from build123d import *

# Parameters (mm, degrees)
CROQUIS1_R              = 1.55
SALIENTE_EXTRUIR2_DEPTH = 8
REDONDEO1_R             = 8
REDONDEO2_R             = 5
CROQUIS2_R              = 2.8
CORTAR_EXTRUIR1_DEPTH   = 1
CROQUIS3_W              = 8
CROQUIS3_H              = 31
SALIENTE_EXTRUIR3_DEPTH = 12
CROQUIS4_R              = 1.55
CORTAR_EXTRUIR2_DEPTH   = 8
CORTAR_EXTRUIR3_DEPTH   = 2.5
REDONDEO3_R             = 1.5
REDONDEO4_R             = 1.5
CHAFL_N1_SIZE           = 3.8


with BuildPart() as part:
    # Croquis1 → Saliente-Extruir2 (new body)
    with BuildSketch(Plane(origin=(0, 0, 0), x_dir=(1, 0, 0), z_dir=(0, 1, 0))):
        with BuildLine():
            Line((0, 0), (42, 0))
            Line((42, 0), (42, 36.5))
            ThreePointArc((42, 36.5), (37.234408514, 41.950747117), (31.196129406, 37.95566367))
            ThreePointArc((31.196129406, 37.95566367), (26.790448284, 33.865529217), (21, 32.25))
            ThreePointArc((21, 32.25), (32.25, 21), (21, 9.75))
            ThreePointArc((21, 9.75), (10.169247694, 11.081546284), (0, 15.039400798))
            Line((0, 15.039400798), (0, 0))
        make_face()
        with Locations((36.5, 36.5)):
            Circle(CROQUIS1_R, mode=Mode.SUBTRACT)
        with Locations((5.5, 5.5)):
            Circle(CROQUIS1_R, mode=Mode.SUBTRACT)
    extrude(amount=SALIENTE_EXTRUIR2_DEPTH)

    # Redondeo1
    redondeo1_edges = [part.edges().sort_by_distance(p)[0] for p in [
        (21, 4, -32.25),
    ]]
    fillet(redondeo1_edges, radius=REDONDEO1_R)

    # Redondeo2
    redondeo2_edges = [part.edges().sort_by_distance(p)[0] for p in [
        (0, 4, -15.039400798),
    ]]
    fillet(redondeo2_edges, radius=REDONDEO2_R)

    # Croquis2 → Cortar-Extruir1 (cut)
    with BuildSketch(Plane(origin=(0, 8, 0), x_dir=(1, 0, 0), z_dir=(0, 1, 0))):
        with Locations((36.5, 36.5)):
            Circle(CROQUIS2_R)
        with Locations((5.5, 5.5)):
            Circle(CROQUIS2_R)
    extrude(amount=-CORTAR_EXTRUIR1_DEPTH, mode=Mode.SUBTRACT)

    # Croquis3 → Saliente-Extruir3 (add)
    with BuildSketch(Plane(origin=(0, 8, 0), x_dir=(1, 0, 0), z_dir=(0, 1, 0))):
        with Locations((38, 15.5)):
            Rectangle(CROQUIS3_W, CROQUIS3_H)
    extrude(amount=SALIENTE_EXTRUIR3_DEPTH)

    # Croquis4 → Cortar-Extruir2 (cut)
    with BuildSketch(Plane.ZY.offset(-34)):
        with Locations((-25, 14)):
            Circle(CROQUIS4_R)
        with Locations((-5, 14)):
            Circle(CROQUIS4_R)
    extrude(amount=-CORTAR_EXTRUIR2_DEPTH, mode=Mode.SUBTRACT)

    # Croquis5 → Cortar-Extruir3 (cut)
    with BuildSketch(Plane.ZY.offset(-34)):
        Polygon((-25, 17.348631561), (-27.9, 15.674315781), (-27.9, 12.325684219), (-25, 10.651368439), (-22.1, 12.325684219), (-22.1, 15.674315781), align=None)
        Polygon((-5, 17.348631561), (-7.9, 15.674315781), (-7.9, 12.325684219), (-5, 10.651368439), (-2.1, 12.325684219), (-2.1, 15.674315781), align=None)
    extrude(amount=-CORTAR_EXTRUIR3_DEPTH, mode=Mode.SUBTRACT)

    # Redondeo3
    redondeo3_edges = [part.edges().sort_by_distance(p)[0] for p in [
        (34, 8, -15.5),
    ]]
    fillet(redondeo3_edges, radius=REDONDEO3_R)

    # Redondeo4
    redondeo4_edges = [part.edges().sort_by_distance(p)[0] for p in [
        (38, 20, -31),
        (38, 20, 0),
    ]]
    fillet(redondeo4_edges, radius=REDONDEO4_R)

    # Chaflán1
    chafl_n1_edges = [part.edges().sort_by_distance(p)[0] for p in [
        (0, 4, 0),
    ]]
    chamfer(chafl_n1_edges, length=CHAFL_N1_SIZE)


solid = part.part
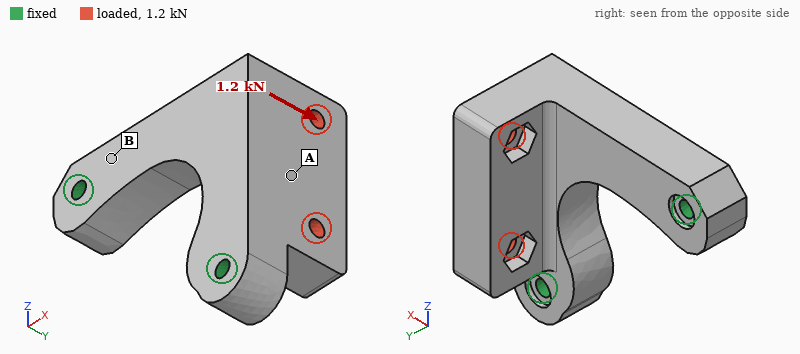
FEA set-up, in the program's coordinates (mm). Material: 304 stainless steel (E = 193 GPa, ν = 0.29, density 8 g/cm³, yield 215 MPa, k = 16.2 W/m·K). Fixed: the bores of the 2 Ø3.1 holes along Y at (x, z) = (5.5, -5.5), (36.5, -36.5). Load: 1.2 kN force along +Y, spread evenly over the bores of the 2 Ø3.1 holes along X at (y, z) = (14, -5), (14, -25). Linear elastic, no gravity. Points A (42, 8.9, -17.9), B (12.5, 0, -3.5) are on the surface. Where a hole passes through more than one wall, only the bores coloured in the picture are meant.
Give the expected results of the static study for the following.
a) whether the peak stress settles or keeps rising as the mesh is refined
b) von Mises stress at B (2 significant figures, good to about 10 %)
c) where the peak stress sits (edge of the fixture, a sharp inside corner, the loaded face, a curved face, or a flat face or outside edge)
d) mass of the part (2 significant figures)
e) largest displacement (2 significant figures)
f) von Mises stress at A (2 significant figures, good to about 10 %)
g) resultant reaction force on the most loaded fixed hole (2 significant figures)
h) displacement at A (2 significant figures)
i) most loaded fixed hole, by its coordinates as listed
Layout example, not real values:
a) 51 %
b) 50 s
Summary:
a) keeps rising
b) 60 MPa
c) edge of the fixture
d) 72 g
e) 49 µm
f) 23 MPa
g) 840 N
h) 23 µm
i) (36.5, -36.5)
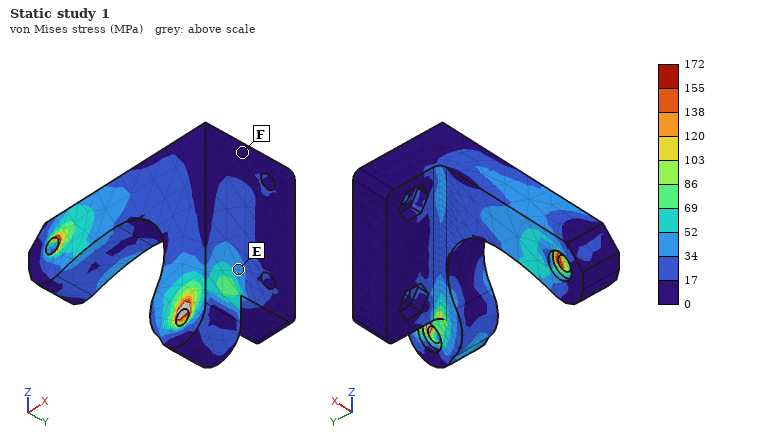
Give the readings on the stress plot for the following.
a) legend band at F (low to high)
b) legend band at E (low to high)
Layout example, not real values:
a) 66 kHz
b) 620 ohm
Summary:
a) 0 to 17 MPa
b) 34 to 52 MPa
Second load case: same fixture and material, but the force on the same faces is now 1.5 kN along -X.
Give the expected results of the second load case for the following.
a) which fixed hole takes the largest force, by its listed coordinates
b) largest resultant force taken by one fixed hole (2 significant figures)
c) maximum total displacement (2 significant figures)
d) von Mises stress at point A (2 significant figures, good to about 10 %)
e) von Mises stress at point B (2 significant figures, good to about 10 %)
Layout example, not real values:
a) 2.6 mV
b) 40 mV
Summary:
a) (5.5, -5.5)
b) 1.0 kN
c) 34 µm
d) 20 MPa
e) 15 MPa
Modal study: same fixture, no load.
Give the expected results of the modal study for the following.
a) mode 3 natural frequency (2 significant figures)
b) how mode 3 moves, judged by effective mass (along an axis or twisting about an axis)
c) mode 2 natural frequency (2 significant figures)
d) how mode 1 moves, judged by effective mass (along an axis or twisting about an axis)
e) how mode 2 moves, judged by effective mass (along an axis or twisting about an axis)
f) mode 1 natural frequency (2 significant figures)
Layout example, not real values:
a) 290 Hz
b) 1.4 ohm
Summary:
a) 20 kHz
b) along Z
c) 11 kHz
d) along Y
e) along X
f) 4700 Hz
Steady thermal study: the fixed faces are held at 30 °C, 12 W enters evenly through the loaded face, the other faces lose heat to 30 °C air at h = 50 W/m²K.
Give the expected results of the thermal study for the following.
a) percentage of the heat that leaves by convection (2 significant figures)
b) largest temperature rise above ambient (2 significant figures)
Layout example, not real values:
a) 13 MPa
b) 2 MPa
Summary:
a) 48 %
b) 73 K
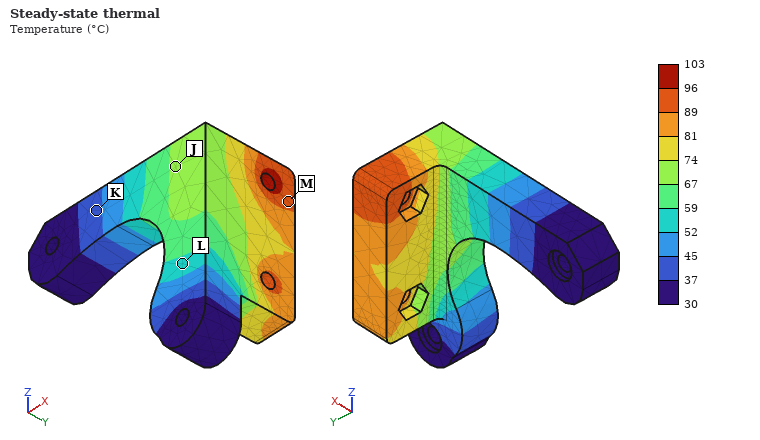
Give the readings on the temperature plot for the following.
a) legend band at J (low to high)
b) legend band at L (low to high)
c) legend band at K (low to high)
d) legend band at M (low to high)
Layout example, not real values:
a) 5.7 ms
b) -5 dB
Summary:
a) 67 to 74 °C
b) 52 to 59 °C
c) 37 to 45 °C
d) 89 to 96 °C
